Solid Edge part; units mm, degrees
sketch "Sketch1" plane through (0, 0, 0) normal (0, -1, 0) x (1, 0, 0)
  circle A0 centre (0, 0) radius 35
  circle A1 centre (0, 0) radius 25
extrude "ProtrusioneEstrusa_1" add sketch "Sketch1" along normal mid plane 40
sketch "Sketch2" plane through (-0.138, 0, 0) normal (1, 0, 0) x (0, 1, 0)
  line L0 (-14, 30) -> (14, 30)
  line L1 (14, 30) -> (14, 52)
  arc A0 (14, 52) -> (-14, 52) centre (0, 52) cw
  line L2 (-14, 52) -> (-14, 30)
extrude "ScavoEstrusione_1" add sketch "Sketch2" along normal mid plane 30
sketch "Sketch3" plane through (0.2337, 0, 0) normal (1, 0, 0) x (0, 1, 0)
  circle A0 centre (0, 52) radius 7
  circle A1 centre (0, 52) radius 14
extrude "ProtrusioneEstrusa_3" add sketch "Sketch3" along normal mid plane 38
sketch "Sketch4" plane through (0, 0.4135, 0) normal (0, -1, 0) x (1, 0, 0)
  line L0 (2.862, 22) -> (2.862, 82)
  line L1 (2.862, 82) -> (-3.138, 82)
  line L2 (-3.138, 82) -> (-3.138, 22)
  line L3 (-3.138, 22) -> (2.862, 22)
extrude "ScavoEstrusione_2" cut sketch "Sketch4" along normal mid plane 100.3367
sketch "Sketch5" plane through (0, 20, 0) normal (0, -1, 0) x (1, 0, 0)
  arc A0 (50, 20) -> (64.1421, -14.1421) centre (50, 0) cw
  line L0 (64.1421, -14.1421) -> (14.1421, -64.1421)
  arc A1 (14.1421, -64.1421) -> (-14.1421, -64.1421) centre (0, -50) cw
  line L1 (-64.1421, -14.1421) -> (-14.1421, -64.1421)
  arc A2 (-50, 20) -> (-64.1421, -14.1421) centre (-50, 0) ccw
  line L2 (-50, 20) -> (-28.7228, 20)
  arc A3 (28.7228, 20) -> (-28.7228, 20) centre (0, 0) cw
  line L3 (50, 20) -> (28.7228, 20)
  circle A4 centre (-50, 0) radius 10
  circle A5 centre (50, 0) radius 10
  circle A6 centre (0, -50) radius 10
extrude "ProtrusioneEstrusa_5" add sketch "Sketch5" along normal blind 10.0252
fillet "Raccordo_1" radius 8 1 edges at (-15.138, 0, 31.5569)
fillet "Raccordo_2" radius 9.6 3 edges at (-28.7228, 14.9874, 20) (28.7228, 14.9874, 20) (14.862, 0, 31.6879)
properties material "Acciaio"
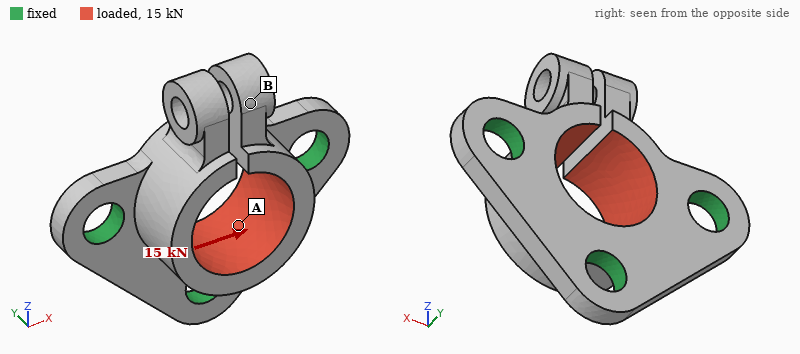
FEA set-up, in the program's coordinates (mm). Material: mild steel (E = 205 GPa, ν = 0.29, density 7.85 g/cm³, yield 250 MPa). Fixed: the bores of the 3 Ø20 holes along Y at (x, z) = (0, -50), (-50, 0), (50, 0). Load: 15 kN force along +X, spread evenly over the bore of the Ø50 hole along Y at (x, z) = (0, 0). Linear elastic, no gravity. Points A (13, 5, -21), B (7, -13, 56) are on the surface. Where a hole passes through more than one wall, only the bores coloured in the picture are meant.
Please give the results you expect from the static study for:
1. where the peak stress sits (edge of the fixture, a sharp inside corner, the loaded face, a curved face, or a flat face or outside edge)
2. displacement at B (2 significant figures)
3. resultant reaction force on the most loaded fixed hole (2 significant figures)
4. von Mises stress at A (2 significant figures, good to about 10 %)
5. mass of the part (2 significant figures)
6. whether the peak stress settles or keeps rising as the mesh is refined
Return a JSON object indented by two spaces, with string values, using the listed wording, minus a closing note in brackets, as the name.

{
  "where the peak stress sits": "a sharp inside corner",
  "displacement at B": "80 µm",
  "resultant reaction force on the most loaded fixed hole": "6.2 kN",
  "von Mises stress at A": "35 MPa",
  "mass of the part": "1.1 kg",
  "whether the peak stress settles or keeps rising as the mesh is refined": "keeps rising"
}
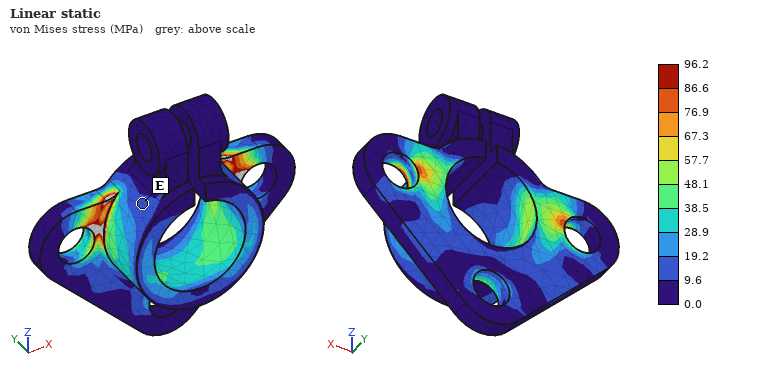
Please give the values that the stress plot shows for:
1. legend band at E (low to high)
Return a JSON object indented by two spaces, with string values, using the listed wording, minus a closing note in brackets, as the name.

{
  "legend band at E": "9.6 to 19.2 MPa"
}
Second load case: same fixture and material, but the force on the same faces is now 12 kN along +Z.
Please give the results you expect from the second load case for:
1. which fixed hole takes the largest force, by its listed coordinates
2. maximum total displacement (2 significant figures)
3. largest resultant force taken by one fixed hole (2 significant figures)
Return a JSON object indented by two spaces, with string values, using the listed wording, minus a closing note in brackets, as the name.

{
  "which fixed hole takes the largest force, by its listed coordinates": "(0, -50)",
  "maximum total displacement": "52 µm",
  "largest resultant force taken by one fixed hole": "6.1 kN"
}
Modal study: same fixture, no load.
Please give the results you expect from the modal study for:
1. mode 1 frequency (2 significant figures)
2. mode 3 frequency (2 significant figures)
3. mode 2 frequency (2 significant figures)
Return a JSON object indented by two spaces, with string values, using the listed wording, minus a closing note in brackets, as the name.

{
  "mode 1 frequency": "1900 Hz",
  "mode 3 frequency": "2500 Hz",
  "mode 2 frequency": "1900 Hz"
}
